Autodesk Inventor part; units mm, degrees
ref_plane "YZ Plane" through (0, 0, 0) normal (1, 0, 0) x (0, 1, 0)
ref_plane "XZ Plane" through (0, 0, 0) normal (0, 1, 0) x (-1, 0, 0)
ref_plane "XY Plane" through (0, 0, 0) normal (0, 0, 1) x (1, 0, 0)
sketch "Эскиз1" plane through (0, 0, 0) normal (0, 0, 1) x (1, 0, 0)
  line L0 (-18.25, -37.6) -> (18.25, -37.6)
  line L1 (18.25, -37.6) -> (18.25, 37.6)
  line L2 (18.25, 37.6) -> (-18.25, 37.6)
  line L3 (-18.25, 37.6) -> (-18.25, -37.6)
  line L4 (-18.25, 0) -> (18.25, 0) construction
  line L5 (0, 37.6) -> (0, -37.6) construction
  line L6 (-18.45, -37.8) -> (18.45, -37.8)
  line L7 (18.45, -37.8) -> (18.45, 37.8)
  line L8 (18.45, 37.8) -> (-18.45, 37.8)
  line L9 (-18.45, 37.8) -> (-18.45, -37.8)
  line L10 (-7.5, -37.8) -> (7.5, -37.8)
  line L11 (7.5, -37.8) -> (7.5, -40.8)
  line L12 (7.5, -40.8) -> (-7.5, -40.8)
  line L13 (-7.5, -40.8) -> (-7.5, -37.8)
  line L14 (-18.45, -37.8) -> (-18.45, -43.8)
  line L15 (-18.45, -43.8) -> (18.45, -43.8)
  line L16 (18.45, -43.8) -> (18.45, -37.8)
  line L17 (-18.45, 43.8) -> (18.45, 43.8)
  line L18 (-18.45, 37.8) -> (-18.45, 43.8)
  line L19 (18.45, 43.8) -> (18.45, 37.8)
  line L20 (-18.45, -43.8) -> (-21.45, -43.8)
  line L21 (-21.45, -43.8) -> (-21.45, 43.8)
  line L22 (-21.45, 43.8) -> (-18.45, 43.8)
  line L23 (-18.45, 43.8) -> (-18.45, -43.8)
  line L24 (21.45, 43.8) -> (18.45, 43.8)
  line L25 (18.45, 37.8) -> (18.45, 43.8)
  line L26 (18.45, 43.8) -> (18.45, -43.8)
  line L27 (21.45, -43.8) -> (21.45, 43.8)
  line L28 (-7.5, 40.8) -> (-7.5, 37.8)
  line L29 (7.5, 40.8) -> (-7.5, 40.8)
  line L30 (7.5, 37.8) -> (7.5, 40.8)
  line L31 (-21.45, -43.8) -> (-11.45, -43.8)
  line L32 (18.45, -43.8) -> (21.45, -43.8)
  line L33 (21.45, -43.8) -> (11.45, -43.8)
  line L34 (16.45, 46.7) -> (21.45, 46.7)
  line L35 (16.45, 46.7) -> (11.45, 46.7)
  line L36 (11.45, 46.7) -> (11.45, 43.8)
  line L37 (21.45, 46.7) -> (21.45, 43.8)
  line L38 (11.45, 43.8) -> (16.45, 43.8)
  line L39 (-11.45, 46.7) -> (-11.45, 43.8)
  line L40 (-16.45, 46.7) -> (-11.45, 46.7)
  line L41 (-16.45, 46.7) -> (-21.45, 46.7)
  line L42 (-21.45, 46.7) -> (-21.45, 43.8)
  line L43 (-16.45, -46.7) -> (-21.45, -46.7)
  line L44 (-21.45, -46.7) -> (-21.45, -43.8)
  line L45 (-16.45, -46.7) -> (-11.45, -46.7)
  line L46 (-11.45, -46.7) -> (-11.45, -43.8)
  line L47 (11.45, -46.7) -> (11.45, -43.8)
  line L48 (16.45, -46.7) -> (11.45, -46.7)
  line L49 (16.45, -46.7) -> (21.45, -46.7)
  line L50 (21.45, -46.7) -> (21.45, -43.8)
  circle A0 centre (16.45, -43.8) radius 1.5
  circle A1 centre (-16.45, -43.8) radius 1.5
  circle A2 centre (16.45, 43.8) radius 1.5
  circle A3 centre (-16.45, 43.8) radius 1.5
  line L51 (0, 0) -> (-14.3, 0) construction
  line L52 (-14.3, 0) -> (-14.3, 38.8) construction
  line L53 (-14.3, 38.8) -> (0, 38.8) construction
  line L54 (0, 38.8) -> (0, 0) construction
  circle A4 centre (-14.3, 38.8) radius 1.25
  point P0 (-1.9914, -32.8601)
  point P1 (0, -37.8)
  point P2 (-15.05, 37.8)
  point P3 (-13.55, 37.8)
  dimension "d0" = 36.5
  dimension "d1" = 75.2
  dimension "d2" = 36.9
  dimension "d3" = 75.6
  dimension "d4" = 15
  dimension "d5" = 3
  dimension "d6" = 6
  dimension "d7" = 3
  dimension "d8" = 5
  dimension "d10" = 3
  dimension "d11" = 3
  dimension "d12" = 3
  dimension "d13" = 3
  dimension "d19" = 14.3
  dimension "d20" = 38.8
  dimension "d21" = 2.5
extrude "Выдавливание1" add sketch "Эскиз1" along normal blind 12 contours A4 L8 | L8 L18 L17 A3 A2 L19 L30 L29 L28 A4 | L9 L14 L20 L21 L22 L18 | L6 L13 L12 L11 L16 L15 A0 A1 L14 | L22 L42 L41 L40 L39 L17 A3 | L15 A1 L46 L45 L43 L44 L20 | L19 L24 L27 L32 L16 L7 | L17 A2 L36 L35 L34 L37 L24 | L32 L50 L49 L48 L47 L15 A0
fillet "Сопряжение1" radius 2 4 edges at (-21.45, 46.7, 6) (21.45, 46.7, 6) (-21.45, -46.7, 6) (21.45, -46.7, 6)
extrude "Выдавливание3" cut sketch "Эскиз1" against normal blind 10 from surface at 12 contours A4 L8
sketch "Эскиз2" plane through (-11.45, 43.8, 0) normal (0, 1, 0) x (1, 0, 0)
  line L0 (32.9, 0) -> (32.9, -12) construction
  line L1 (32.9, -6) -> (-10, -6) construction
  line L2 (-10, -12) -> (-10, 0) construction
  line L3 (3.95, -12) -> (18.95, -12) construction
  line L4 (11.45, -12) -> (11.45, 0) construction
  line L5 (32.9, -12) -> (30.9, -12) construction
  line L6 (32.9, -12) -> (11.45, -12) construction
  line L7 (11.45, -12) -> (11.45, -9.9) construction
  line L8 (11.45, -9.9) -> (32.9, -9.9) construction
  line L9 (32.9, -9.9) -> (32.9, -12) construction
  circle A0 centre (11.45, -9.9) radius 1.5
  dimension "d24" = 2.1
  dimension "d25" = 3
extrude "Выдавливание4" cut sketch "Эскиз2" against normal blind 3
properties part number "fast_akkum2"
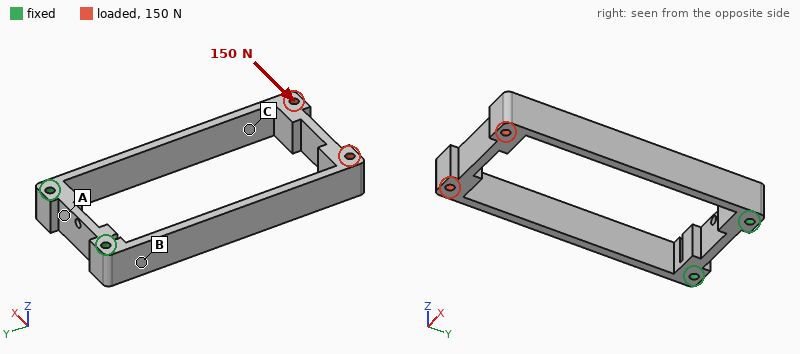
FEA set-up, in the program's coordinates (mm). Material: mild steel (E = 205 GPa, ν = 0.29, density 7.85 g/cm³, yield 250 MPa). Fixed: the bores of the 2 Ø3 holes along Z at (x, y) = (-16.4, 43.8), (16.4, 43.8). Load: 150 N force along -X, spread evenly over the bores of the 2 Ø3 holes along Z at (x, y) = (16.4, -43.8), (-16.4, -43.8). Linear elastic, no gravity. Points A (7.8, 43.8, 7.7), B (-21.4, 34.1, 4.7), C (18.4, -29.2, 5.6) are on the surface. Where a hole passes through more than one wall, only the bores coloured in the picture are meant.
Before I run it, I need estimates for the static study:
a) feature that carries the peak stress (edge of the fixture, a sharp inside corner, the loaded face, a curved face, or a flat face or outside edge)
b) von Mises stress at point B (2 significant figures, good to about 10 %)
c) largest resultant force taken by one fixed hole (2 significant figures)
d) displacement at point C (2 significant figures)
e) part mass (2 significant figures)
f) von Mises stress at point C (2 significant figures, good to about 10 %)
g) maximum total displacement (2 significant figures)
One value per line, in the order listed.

a flat face or outside edge
140 MPa
210 N
0.55 mm
90 g
120 MPa
0.59 mm
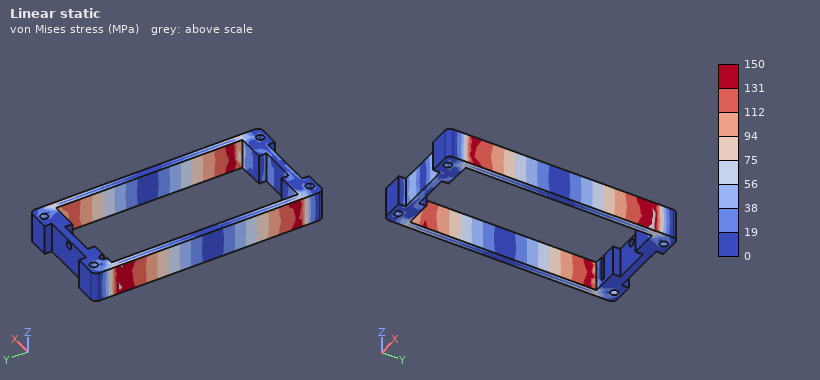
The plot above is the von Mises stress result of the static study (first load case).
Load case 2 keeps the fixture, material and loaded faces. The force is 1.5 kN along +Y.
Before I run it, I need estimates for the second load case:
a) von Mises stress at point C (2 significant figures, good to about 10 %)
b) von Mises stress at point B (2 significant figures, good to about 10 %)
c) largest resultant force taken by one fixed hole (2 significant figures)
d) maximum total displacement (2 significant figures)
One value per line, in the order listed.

59 MPa
38 MPa
760 N
53 µm
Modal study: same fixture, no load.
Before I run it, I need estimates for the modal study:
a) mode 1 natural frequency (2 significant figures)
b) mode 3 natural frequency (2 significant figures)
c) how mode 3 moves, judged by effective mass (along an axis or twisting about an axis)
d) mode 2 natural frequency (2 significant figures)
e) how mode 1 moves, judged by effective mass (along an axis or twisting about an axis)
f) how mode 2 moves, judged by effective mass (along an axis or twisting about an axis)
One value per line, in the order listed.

410 Hz
1400 Hz
twisting about Y
810 Hz
along X
along Z
